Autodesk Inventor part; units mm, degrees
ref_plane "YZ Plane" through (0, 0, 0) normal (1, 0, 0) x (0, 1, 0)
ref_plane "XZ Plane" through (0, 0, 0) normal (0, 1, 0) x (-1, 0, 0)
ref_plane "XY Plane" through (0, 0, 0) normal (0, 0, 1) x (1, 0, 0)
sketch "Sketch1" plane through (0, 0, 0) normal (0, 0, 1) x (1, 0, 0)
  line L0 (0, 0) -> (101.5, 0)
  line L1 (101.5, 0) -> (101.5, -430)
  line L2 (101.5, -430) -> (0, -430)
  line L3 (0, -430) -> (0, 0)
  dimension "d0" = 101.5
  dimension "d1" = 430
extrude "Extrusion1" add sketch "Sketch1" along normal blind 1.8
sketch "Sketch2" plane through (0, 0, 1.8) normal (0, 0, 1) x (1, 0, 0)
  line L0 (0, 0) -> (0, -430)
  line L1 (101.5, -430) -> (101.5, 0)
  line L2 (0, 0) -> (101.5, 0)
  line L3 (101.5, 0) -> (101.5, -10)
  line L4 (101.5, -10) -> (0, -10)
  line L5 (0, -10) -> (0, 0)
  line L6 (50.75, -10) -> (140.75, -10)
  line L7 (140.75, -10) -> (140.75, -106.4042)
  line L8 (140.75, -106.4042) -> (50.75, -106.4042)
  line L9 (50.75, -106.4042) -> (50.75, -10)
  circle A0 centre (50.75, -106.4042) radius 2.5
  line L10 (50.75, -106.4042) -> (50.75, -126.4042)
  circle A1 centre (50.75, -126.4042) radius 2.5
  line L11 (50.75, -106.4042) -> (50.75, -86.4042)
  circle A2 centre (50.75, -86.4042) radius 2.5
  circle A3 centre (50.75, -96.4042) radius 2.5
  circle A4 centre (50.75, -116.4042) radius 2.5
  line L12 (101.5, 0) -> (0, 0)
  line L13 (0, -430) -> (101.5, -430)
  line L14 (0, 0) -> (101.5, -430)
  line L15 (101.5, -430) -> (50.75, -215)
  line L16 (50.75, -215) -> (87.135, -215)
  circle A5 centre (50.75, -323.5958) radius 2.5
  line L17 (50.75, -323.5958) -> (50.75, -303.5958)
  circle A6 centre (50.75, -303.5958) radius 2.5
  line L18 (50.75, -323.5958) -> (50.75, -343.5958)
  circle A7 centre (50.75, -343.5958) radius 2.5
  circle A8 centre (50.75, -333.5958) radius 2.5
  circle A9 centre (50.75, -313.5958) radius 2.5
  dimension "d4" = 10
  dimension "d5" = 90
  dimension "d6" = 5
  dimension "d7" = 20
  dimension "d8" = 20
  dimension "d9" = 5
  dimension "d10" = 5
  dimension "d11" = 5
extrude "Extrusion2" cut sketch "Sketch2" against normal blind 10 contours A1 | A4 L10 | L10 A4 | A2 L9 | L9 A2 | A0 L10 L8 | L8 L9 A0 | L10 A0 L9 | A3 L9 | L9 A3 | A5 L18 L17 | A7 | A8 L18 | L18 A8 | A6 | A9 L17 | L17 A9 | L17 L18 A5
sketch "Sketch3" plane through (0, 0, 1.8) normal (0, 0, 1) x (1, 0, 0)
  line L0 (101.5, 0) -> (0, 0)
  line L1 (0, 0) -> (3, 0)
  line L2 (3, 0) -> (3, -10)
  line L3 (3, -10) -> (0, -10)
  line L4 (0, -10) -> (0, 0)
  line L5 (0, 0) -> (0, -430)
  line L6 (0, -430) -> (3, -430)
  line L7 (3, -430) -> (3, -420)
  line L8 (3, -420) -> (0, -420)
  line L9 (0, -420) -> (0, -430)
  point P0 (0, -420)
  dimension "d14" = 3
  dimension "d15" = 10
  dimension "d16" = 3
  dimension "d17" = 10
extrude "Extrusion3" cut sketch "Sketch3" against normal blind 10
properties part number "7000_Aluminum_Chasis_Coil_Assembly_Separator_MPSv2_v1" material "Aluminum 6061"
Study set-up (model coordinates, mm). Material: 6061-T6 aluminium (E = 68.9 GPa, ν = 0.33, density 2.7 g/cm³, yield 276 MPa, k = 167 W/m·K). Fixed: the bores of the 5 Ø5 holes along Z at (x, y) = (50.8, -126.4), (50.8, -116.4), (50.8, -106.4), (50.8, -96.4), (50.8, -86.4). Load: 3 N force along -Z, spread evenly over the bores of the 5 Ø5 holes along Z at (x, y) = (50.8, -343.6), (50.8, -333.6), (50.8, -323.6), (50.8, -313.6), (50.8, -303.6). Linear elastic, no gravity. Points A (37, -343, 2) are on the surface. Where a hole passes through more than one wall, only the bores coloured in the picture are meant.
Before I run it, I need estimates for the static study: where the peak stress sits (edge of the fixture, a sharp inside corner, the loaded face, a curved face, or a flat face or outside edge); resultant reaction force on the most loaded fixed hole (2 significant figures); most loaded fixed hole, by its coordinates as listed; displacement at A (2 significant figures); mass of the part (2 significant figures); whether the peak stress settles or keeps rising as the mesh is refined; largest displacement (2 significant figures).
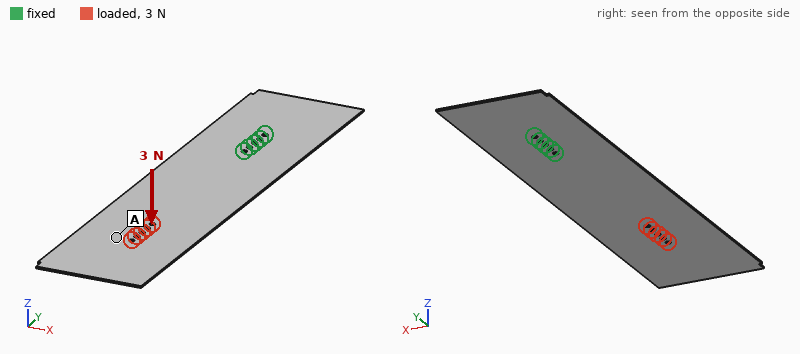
edge of the fixture
23 N
(50.8, -126.4)
2.7 mm
210 g
keeps rising
4.2 mm
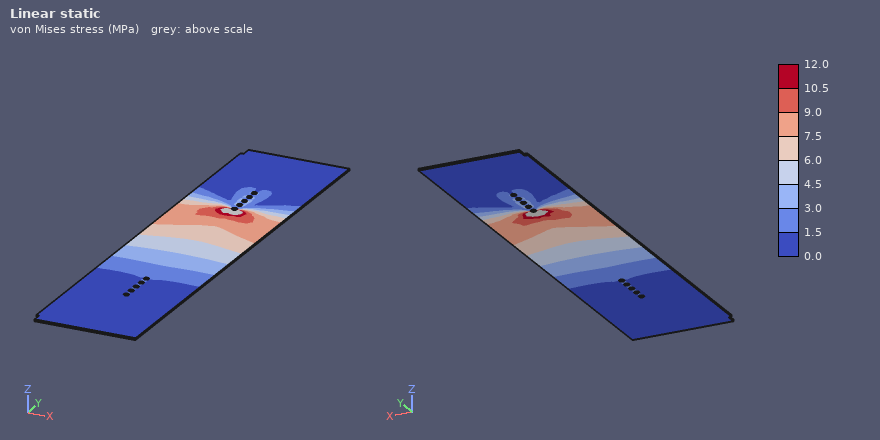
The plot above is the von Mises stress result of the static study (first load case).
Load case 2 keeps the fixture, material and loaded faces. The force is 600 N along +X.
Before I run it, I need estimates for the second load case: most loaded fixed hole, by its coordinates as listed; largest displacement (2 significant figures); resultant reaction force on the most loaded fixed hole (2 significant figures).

(50.8, -126.4)
0.70 mm
2.9 kN
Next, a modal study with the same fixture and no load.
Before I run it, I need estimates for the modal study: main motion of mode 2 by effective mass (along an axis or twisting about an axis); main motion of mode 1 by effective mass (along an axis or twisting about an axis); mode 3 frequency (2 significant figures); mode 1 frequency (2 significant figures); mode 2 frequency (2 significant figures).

twisting about Y
along Z
97 Hz
16 Hz
89 Hz
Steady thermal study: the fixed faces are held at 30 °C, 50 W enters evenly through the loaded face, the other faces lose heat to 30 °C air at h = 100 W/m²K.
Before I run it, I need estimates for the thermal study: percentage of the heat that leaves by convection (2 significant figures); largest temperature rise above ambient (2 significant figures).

100 %
46 K
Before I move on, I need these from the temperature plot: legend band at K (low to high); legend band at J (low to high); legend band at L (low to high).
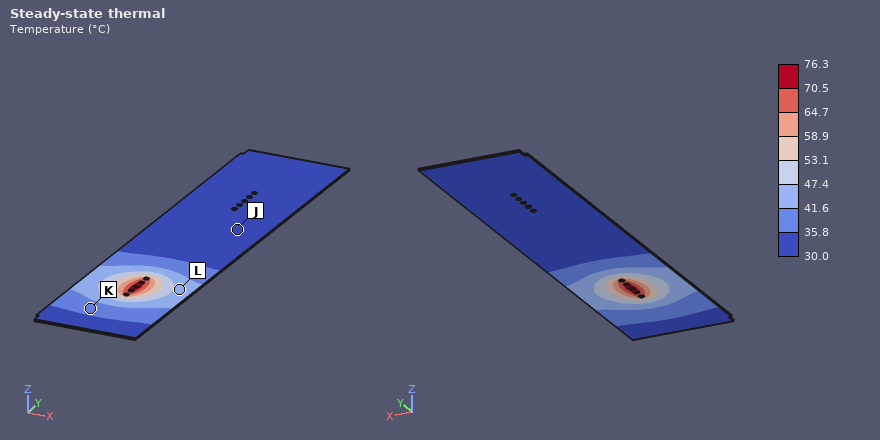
35.8 to 41.6 °C
30.0 to 35.8 °C
41.6 to 47.4 °C
